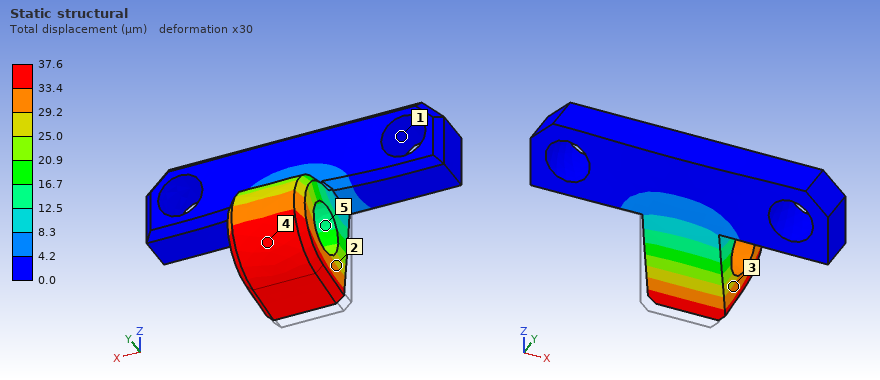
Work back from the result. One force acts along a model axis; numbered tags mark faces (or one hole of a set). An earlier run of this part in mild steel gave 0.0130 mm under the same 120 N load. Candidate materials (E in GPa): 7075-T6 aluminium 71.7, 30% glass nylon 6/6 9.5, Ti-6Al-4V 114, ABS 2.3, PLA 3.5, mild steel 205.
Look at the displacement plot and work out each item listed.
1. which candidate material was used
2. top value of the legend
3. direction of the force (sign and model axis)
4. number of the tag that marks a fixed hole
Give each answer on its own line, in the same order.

7075-T6 aluminium
37.6 µm
+Y
1
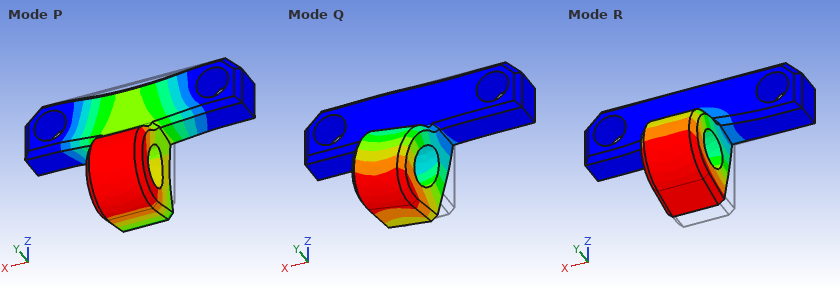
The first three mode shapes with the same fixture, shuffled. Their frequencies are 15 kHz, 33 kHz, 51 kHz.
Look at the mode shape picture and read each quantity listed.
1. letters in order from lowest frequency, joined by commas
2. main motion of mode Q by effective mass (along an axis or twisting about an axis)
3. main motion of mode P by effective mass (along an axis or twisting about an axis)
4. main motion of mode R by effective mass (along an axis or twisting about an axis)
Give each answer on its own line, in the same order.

R, Q, P
along X
along Z
along Y
